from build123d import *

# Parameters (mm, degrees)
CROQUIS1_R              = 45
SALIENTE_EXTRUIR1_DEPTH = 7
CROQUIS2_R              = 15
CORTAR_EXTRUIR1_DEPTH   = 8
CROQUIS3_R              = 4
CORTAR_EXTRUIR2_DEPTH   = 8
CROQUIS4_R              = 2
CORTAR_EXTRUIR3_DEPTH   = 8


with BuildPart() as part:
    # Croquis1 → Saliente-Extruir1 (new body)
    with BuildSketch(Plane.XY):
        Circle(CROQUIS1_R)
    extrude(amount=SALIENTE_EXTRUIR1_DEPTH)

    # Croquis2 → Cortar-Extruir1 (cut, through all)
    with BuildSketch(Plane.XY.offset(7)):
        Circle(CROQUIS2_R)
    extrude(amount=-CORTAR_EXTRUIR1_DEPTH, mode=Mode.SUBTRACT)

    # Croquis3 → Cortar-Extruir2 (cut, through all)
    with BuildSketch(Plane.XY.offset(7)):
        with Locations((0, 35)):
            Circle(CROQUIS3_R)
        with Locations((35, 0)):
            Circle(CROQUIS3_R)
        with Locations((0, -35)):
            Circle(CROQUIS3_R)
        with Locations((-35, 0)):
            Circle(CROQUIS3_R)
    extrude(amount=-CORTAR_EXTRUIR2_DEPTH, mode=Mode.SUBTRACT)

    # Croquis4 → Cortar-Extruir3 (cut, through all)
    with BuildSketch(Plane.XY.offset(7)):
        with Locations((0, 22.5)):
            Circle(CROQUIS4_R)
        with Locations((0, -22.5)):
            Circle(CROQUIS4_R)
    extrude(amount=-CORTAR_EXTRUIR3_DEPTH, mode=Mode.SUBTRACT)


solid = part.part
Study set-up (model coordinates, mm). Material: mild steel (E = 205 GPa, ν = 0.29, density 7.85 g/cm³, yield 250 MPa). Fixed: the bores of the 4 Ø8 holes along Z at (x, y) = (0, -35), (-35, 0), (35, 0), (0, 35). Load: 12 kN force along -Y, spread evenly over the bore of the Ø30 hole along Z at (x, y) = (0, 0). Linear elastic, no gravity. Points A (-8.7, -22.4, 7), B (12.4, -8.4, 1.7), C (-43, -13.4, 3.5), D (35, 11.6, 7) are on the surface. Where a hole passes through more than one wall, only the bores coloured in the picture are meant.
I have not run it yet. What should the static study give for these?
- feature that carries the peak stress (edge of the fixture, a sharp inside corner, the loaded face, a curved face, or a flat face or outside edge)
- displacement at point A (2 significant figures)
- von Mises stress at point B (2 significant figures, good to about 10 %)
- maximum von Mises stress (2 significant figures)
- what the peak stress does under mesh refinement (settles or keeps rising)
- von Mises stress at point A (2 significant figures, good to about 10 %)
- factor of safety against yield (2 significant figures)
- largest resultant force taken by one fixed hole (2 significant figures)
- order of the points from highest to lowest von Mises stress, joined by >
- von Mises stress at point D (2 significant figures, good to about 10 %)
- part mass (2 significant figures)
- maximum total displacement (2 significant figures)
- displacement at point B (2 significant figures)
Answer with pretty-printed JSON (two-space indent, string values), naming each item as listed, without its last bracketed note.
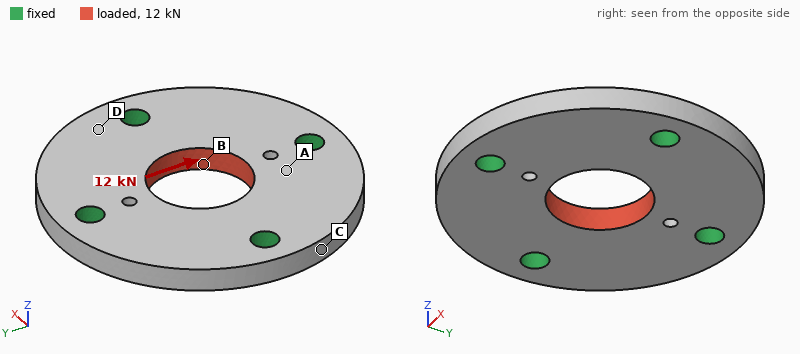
{
  "feature that carries the peak stress": "a curved face",
  "displacement at point A": "1.8 µm",
  "von Mises stress at point B": "28 MPa",
  "maximum von Mises stress": "77 MPa",
  "what the peak stress does under mesh refinement": "settles",
  "von Mises stress at point A": "18 MPa",
  "factor of safety against yield": "3.2",
  "largest resultant force taken by one fixed hole": "3.5 kN",
  "order of the points from highest to lowest von Mises stress, joined by >": "B > A > D > C",
  "von Mises stress at point D": "10 MPa",
  "part mass": "300 g",
  "maximum total displacement": "3.2 µm",
  "displacement at point B": "3.0 µm"
}
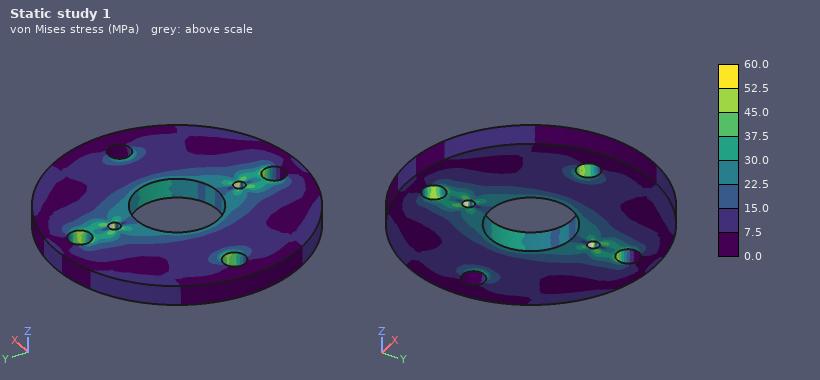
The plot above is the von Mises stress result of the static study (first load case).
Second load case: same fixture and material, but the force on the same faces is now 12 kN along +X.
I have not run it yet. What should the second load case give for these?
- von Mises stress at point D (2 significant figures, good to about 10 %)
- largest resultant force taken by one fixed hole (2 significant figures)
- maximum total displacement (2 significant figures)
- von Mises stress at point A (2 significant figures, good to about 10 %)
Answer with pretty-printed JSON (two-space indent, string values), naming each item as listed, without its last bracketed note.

{
  "von Mises stress at point D": "10 MPa",
  "largest resultant force taken by one fixed hole": "3.6 kN",
  "maximum total displacement": "3.1 µm",
  "von Mises stress at point A": "11 MPa"
}
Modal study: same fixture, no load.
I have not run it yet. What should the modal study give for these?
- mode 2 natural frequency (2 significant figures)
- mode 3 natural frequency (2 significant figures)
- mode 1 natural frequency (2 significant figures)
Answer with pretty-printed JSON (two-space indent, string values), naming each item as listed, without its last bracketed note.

{
  "mode 2 natural frequency": "11 kHz",
  "mode 3 natural frequency": "11 kHz",
  "mode 1 natural frequency": "11 kHz"
}
